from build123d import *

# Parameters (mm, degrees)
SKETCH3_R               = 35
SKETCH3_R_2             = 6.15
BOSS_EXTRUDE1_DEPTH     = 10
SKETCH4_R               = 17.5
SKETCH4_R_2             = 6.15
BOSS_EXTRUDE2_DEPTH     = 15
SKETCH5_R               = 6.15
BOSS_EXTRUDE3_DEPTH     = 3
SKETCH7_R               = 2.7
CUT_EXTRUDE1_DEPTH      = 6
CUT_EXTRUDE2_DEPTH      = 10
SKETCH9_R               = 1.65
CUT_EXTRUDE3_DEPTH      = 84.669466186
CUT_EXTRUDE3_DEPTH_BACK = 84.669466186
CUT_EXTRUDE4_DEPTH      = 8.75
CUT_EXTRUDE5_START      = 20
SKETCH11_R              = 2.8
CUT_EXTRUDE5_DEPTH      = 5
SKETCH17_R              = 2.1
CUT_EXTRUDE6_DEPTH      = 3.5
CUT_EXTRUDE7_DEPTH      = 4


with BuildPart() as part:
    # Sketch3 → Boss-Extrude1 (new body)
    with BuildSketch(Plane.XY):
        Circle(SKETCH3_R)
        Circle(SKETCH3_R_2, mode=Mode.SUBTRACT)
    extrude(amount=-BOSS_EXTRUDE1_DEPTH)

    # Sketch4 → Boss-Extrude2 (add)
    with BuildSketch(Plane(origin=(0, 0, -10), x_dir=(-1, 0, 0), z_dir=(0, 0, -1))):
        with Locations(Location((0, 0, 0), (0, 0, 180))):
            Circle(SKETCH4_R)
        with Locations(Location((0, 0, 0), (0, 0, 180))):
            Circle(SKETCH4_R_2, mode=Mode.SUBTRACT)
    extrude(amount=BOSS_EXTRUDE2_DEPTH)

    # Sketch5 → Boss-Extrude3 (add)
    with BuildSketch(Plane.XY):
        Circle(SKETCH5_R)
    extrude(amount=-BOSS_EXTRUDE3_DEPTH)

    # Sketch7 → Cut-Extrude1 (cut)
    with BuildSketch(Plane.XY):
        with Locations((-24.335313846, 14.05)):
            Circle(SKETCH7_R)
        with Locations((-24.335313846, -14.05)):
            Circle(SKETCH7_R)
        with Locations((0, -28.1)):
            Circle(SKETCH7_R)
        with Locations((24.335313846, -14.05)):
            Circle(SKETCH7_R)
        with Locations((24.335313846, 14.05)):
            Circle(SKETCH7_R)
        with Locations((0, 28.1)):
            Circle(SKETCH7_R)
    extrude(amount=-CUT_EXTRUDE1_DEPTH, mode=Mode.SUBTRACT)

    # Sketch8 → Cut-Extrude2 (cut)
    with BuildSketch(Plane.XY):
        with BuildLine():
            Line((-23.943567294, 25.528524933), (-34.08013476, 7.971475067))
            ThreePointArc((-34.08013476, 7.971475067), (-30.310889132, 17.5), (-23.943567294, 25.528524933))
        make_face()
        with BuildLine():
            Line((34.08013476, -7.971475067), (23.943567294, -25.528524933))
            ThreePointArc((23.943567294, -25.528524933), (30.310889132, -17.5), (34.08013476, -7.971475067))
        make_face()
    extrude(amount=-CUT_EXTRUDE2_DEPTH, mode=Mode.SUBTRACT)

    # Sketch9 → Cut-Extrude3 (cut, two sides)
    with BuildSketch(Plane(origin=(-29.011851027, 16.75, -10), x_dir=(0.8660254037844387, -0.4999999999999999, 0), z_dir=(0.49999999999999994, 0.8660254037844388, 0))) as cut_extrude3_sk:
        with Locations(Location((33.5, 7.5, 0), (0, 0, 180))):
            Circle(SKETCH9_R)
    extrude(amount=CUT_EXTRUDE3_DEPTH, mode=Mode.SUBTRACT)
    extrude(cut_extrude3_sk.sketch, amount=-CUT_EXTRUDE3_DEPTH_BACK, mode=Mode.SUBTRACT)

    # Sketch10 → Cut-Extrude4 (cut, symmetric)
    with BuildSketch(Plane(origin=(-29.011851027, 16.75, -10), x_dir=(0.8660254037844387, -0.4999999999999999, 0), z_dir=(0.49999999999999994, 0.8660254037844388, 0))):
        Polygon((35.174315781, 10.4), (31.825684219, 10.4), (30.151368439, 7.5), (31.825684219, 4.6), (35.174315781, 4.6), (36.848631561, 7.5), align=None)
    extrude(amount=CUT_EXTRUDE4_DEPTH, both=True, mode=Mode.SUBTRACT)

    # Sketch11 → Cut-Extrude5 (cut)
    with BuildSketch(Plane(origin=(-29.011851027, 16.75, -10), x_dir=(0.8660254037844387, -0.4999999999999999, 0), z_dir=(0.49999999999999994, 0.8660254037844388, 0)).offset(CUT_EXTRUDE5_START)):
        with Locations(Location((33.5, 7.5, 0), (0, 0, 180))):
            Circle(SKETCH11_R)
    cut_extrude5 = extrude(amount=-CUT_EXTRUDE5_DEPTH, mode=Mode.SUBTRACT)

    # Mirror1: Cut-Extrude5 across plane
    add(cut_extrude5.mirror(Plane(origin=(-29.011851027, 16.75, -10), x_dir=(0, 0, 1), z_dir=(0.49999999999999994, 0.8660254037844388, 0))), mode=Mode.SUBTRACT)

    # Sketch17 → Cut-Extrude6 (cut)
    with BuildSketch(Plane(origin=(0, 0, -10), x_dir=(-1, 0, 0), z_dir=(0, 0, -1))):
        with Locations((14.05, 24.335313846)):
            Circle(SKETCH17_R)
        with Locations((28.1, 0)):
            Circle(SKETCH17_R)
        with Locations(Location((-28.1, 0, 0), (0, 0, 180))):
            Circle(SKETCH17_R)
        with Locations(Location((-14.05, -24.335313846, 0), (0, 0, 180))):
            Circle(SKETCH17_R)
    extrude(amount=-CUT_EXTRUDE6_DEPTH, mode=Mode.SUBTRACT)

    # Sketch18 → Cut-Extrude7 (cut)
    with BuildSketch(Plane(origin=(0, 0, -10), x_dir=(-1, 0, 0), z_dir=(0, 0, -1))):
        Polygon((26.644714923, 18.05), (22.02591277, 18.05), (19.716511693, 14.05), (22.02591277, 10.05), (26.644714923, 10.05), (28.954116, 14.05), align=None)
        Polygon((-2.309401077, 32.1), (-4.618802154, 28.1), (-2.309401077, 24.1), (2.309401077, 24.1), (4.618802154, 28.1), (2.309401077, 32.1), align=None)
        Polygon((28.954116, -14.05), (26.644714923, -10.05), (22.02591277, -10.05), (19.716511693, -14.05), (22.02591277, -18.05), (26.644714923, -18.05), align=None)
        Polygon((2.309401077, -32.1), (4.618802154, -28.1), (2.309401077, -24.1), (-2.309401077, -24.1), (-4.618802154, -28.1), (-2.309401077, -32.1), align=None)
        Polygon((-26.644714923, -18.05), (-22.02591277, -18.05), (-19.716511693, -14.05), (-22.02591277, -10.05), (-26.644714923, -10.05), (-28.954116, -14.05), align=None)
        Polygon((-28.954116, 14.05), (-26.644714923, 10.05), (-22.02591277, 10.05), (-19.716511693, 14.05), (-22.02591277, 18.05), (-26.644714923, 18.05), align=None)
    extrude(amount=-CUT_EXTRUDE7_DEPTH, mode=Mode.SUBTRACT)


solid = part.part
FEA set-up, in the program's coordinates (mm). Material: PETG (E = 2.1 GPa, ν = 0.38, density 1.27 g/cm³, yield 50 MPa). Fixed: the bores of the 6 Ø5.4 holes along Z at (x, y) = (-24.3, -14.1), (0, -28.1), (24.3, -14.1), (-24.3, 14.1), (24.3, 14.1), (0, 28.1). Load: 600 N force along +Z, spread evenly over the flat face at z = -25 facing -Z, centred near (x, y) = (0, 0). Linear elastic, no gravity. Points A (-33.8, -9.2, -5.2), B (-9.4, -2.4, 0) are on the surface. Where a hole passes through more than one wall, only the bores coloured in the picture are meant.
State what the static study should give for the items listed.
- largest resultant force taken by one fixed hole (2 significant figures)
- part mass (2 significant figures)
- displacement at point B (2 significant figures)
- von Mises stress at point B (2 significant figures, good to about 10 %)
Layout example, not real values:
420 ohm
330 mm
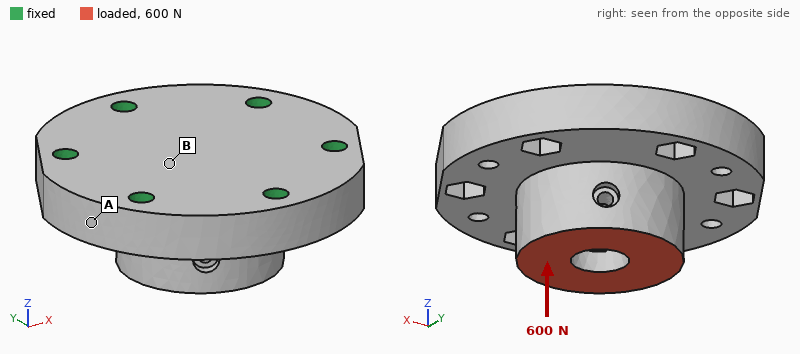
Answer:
120 N
60 g
23 µm
0.94 MPa
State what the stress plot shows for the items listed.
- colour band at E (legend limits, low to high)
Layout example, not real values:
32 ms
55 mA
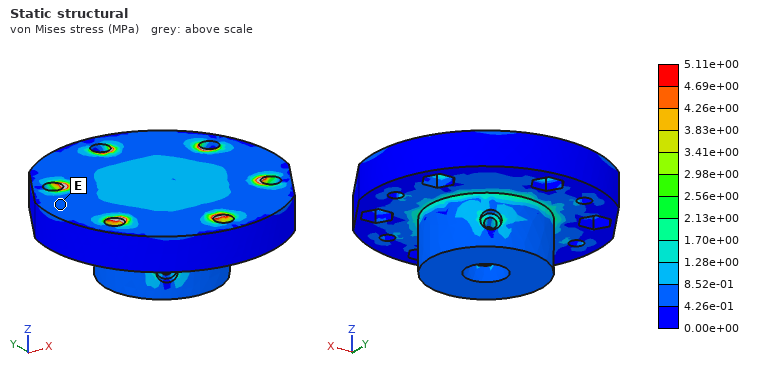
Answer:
4.26e-01 to 8.52e-01 MPa
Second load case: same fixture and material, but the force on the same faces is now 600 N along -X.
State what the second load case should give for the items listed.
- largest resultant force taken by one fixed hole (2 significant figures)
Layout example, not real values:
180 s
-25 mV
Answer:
200 N
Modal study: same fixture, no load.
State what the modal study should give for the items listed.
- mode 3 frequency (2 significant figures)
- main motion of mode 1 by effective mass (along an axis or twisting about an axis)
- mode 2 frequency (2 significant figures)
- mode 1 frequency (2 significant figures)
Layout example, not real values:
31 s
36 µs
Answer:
5300 Hz
along Z
5300 Hz
4600 Hz
